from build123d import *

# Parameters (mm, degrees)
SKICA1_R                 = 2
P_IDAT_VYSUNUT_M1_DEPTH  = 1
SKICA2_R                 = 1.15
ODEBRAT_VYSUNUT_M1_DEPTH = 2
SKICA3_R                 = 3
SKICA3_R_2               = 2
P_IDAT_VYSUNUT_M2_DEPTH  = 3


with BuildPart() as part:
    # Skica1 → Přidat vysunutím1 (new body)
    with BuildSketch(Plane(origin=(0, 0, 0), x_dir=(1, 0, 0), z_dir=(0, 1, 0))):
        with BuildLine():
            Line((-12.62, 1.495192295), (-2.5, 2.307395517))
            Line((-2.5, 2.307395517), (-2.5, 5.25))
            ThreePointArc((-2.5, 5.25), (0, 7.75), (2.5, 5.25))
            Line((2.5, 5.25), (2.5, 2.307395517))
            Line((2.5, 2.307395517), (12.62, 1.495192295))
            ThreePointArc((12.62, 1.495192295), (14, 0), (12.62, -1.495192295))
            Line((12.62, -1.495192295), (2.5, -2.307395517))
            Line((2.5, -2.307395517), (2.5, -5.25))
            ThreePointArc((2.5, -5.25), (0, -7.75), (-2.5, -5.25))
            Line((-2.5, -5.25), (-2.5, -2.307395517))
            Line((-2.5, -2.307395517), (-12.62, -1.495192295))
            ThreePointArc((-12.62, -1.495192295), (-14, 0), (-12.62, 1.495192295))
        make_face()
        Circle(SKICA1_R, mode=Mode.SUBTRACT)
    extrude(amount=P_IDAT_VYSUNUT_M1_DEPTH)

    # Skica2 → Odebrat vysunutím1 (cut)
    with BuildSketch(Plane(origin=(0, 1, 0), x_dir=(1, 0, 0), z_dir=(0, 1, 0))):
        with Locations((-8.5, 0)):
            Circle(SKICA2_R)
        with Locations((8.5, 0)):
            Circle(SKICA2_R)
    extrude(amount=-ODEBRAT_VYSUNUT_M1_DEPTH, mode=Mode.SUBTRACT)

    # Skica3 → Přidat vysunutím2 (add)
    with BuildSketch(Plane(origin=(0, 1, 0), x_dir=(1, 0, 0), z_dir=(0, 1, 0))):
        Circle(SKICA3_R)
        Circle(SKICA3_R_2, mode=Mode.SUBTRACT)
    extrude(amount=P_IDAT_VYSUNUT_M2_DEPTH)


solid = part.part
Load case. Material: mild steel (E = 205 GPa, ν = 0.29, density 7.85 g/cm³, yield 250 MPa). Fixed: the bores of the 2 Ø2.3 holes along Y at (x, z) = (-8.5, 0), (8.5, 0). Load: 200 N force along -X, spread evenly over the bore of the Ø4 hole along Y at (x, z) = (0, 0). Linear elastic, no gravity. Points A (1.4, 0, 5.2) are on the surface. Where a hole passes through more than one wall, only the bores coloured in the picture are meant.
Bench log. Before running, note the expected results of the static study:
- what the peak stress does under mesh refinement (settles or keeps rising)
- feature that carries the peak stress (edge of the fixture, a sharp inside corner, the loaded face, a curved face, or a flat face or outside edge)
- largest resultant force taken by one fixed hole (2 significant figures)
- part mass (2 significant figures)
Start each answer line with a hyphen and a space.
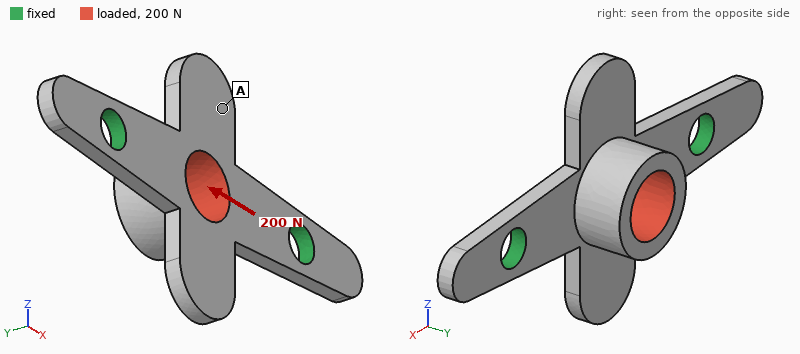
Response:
- keeps rising
- edge of the fixture
- 100 N
- 1.4 g
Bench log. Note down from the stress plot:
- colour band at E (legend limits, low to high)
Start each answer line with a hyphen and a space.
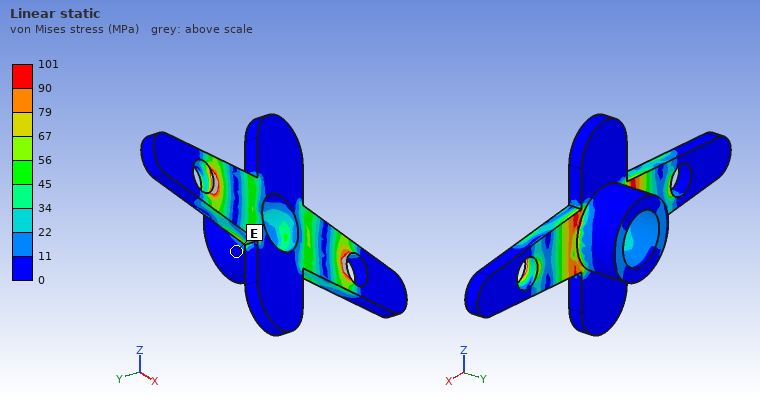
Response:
- 0 to 11 MPa
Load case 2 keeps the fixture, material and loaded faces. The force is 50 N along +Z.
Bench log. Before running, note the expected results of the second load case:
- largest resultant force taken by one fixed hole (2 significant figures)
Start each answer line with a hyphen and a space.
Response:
- 25 N
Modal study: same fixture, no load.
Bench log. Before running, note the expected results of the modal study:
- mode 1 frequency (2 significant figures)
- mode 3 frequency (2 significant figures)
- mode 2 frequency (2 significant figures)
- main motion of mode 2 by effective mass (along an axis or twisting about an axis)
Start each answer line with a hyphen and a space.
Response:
- 8900 Hz
- 35 kHz
- 14 kHz
- along Y
